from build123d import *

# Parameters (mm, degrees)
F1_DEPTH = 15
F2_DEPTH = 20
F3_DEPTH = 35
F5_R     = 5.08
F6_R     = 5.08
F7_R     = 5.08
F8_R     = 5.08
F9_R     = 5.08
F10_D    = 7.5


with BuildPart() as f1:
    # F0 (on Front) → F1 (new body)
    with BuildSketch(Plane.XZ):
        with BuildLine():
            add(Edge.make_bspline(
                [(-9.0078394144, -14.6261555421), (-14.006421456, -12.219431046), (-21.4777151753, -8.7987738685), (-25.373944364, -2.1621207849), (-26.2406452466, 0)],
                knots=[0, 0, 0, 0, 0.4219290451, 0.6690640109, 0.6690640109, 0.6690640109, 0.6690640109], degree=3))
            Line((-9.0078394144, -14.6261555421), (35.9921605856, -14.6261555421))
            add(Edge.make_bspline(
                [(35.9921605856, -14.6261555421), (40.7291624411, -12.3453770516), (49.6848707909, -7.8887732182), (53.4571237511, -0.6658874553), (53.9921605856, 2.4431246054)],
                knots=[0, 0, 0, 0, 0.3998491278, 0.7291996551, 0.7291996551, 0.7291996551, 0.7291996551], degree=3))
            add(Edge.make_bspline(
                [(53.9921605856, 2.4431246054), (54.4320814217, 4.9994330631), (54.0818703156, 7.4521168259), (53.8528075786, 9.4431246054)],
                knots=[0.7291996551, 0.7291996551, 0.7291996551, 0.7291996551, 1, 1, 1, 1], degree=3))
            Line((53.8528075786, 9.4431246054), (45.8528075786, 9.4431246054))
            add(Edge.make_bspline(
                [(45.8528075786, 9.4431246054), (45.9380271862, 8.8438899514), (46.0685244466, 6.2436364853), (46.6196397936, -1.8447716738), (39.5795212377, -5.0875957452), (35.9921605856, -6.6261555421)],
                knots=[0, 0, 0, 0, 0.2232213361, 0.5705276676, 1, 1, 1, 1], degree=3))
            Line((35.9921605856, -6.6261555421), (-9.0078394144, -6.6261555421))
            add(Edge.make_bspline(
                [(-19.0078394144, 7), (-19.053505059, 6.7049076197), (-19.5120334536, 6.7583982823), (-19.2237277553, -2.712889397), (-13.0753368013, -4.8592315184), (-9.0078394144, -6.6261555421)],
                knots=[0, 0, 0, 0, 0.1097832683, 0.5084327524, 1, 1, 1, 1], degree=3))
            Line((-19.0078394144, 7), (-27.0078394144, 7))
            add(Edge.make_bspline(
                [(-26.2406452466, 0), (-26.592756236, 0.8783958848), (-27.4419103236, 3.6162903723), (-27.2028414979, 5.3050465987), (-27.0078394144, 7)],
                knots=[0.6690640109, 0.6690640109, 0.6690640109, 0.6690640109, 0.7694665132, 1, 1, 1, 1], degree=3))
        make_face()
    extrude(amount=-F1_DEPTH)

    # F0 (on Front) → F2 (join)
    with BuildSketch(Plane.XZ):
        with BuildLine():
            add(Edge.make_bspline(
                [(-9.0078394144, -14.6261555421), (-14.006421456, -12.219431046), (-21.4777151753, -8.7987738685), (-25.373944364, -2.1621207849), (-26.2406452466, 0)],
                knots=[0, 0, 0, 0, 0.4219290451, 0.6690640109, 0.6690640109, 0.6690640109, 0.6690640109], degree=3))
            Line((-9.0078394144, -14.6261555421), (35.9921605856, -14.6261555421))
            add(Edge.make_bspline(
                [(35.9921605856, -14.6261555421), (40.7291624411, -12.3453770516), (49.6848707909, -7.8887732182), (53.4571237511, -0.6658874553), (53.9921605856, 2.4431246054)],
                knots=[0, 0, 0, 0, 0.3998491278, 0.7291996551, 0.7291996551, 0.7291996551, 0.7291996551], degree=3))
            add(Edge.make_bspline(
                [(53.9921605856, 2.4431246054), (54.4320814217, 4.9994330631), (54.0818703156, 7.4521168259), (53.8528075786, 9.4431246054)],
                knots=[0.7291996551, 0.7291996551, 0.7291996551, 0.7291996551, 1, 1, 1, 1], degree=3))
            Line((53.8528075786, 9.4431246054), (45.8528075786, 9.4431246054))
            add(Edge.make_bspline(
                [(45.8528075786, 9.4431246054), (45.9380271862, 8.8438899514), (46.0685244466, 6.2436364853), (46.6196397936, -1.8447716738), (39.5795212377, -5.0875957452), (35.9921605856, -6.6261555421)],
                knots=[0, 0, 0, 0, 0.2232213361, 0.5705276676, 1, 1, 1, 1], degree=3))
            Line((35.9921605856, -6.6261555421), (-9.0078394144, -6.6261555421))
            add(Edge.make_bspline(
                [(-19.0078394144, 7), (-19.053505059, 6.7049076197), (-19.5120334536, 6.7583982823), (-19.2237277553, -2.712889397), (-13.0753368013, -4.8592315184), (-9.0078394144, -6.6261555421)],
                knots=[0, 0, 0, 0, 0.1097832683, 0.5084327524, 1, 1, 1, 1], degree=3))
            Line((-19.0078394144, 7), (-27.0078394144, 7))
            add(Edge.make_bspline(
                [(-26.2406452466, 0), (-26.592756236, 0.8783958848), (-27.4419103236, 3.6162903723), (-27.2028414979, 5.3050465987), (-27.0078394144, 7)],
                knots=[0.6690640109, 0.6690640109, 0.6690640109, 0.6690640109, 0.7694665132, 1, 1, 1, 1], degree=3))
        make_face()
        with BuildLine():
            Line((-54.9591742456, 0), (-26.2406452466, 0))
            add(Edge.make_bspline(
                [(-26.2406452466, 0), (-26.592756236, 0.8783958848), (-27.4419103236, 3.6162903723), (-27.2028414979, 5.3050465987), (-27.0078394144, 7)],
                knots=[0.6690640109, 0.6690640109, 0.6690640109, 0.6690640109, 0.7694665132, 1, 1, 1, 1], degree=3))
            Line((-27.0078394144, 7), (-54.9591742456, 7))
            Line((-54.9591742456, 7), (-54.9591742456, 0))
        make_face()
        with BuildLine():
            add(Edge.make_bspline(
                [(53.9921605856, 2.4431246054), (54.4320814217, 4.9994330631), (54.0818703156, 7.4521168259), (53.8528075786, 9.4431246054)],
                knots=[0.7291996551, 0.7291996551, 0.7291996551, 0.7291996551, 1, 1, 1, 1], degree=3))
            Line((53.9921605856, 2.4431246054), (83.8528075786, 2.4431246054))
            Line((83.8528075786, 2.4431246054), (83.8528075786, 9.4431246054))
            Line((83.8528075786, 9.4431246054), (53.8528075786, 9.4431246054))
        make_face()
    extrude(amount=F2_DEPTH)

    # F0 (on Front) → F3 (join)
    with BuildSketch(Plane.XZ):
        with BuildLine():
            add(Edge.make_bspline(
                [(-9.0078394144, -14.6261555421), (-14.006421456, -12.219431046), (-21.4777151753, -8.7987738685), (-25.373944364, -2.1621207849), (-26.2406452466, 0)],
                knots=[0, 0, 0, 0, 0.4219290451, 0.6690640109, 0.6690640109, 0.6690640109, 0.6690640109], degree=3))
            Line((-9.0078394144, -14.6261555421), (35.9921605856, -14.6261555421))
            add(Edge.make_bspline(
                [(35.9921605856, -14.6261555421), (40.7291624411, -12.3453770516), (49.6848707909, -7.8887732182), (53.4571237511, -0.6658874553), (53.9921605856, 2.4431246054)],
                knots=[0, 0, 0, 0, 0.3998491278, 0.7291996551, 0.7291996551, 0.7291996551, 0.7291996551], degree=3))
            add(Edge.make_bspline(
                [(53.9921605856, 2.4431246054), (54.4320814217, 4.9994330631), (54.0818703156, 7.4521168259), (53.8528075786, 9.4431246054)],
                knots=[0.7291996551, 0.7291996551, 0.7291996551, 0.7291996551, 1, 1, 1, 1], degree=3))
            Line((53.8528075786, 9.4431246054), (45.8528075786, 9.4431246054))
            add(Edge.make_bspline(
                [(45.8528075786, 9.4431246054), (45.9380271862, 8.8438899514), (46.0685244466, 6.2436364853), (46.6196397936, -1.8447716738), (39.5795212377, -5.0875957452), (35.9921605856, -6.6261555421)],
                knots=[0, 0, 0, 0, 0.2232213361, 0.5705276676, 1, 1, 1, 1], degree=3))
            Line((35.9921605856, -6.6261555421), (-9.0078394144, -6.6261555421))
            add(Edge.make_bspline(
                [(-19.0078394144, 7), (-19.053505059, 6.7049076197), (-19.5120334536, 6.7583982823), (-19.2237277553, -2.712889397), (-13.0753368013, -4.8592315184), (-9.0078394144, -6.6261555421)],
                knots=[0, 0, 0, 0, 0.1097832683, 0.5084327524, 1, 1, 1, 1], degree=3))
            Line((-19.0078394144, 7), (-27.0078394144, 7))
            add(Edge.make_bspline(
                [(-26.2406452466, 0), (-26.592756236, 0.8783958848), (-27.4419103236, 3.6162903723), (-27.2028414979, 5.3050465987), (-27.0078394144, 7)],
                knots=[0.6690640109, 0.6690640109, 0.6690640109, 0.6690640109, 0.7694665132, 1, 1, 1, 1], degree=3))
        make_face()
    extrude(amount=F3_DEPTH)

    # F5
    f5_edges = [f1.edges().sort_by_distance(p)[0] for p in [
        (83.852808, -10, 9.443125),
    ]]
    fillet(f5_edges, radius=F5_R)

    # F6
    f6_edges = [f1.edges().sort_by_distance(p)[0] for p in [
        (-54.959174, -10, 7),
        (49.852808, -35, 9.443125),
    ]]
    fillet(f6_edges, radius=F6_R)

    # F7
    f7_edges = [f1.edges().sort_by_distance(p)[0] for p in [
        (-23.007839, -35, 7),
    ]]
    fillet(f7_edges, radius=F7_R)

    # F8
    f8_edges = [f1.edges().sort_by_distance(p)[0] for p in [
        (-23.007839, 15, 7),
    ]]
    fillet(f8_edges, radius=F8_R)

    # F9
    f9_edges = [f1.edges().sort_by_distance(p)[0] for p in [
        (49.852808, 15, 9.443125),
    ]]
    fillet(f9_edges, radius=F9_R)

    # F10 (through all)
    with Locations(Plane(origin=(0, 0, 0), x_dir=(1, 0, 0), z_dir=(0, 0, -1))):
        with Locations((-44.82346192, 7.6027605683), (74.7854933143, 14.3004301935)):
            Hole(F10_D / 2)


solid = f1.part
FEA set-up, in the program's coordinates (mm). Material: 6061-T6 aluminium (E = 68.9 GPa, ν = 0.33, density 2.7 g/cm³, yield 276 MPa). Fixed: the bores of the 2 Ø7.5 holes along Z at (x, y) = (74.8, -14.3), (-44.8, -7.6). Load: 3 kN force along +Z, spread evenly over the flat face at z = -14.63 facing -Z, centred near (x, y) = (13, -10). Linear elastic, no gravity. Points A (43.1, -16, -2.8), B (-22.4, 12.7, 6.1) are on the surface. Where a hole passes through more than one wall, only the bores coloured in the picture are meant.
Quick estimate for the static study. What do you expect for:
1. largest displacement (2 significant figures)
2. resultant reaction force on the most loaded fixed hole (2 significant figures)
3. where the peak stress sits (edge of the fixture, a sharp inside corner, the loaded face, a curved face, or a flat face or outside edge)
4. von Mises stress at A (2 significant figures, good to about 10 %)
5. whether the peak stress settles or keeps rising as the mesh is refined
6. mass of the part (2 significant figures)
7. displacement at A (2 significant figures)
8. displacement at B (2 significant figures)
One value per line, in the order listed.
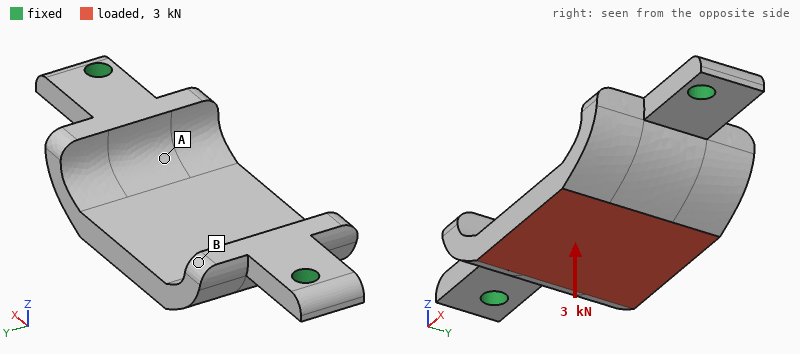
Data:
87 µm
3.1 kN
edge of the fixture
28 MPa
keeps rising
120 g
53 µm
47 µm
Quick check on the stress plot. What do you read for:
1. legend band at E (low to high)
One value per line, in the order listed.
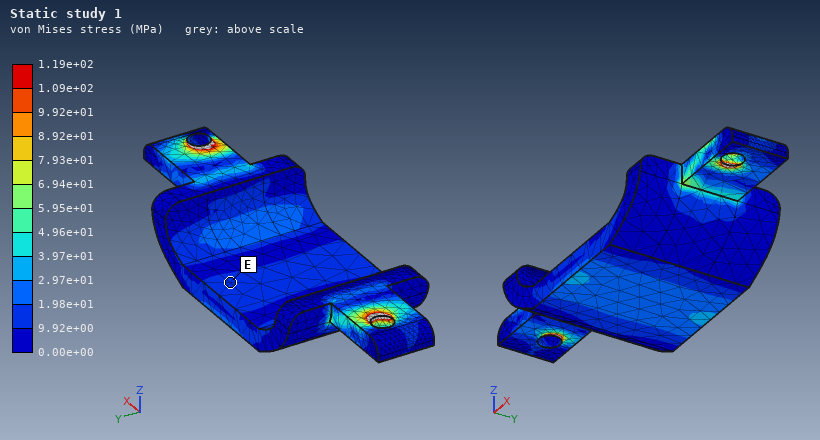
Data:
9.92e+00 to 1.98e+01 MPa
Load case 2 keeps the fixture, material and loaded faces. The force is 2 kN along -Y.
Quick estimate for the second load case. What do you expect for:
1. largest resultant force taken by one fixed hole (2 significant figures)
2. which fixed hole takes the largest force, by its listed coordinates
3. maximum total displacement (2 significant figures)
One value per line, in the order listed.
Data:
1.1 kN
(-44.8, -7.6)
0.30 mm
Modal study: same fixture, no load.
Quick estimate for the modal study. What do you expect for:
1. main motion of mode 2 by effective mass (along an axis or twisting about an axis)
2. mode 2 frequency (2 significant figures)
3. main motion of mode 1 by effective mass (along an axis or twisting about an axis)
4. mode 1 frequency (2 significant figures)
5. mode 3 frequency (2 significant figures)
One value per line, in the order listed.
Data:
along Z
3600 Hz
along Y
1800 Hz
4900 Hz
